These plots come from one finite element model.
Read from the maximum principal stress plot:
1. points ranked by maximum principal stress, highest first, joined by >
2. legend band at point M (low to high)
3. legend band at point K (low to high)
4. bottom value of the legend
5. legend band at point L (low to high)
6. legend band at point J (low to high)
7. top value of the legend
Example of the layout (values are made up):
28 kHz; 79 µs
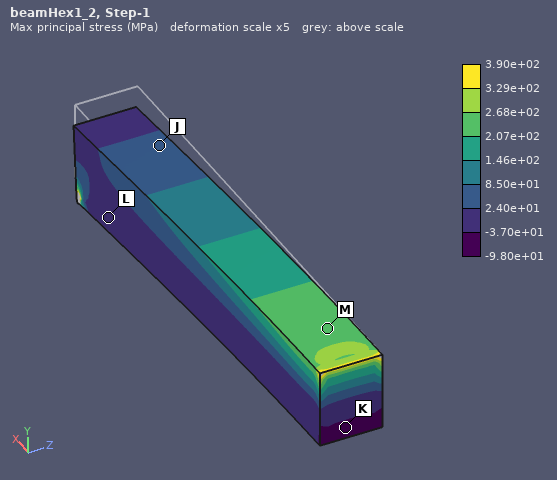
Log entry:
M > J > L > K; 2.07e+02 to 2.68e+02 MPa; -9.80e+01 to -3.70e+01 MPa; -9.80e+01 MPa; -3.70e+01 to 2.40e+01 MPa; 2.40e+01 to 8.50e+01 MPa; 3.90e+02 MPa
